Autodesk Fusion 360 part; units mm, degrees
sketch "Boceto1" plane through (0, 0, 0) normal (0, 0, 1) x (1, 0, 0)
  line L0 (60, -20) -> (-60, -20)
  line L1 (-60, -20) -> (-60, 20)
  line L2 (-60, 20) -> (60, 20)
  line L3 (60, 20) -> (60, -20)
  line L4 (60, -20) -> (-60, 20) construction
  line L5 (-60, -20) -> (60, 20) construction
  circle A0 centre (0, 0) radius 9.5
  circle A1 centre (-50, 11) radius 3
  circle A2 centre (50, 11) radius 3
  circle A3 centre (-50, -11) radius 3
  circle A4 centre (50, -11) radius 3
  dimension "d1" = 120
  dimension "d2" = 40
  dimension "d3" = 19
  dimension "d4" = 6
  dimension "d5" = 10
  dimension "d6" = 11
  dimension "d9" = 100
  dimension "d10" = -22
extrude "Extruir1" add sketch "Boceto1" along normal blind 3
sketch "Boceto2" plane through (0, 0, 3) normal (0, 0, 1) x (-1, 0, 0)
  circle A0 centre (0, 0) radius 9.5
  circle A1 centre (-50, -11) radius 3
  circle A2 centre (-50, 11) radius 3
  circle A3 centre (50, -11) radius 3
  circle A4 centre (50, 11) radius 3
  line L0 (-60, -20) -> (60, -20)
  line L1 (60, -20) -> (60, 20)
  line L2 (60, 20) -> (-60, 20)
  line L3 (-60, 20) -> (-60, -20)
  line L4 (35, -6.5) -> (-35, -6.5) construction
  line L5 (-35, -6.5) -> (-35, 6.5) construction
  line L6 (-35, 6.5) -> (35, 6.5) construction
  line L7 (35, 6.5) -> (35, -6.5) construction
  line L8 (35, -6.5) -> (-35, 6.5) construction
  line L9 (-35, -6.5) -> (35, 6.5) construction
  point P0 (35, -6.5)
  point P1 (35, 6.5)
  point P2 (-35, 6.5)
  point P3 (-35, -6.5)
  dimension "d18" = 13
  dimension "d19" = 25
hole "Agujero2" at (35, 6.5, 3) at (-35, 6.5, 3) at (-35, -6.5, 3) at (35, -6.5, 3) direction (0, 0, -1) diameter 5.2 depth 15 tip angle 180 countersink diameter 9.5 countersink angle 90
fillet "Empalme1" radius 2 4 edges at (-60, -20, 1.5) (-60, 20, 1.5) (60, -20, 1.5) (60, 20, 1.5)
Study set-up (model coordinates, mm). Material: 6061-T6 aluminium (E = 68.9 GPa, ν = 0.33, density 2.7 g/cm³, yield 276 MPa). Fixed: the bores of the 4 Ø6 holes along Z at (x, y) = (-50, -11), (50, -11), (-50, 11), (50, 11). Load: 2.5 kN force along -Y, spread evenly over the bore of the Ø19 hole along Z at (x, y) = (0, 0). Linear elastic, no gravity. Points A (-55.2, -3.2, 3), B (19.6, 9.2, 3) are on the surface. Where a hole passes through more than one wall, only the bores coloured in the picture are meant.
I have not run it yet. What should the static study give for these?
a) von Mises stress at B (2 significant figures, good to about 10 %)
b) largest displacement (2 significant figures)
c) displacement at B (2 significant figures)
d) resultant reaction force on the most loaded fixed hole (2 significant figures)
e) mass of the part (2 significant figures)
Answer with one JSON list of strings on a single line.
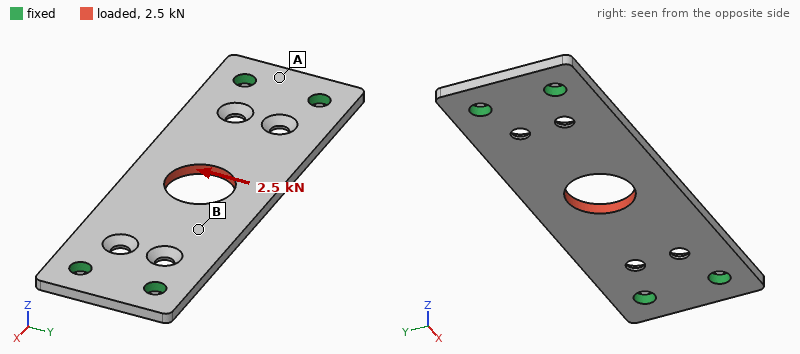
["23 MPa", "42 µm", "29 µm", "1.2 kN", "34 g"]
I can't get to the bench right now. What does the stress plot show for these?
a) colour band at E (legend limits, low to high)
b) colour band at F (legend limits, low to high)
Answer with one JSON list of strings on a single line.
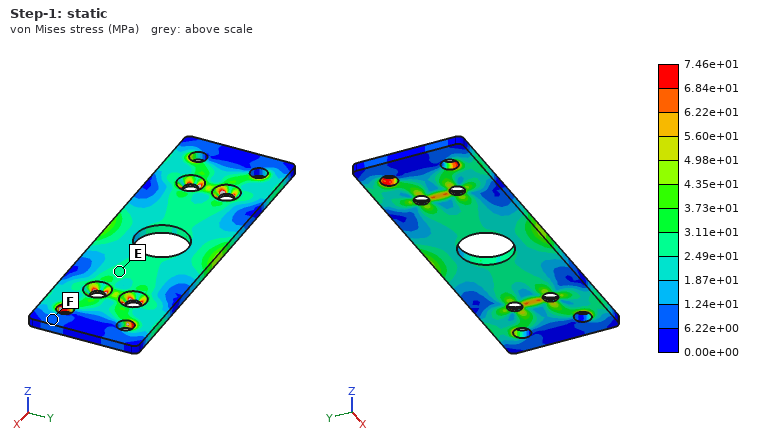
["2.49e+01 to 3.11e+01 MPa", "6.22e+00 to 1.24e+01 MPa"]
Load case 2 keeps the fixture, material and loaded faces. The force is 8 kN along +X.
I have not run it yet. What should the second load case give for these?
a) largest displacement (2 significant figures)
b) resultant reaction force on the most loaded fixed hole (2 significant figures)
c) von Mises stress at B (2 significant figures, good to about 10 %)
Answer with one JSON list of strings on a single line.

["29 µm", "2.0 kN", "36 MPa"]
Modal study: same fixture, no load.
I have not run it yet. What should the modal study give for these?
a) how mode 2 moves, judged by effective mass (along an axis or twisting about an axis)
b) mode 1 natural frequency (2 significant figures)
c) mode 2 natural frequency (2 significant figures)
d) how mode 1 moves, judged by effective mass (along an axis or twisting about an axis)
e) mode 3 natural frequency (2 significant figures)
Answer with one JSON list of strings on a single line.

["twisting about X", "1700 Hz", "2900 Hz", "along Z", "4500 Hz"]
